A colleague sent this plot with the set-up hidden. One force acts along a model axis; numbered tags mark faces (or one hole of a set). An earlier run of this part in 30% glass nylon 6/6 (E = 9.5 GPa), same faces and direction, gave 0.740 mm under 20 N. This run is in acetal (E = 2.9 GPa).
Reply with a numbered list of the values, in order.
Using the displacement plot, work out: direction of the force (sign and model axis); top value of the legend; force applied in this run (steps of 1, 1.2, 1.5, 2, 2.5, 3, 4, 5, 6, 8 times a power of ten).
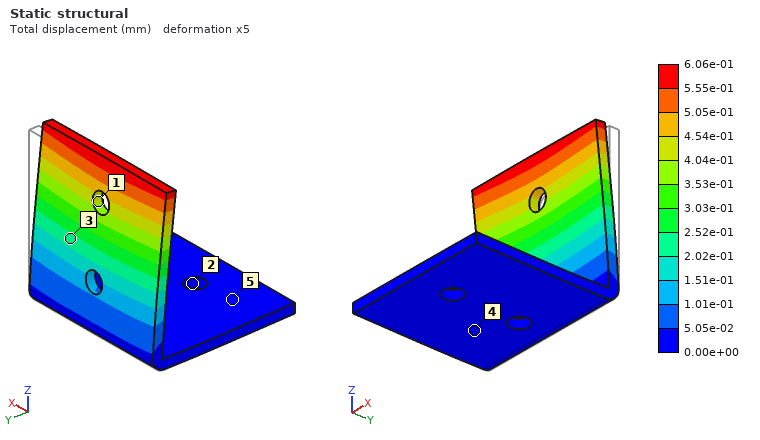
1. -Y
2. 6.06e-01 mm
3. 5 N
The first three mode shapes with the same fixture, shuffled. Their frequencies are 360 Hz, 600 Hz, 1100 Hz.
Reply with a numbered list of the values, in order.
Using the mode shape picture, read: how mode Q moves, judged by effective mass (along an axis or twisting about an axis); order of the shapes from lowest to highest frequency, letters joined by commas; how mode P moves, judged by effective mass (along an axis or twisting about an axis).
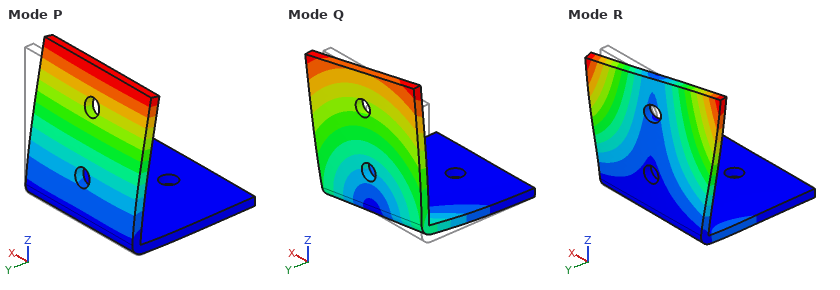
1. along X
2. P, Q, R
3. along Y
